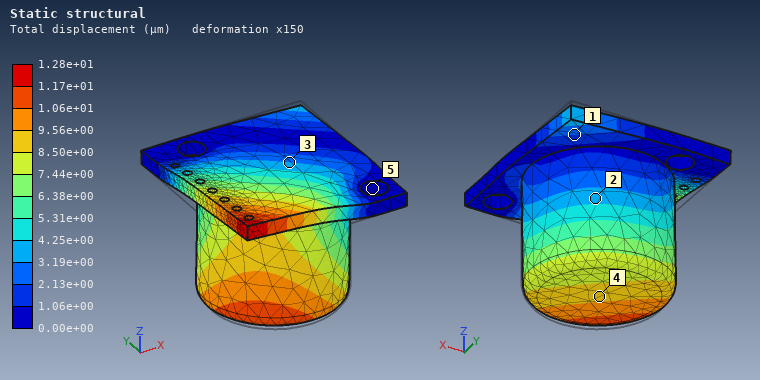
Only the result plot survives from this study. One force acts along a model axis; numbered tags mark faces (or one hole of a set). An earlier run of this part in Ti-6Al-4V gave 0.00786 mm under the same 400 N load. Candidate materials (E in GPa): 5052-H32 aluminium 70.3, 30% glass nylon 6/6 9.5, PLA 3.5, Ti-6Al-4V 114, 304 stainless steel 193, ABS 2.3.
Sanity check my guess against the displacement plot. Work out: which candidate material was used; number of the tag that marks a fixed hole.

5052-H32 aluminium
5
